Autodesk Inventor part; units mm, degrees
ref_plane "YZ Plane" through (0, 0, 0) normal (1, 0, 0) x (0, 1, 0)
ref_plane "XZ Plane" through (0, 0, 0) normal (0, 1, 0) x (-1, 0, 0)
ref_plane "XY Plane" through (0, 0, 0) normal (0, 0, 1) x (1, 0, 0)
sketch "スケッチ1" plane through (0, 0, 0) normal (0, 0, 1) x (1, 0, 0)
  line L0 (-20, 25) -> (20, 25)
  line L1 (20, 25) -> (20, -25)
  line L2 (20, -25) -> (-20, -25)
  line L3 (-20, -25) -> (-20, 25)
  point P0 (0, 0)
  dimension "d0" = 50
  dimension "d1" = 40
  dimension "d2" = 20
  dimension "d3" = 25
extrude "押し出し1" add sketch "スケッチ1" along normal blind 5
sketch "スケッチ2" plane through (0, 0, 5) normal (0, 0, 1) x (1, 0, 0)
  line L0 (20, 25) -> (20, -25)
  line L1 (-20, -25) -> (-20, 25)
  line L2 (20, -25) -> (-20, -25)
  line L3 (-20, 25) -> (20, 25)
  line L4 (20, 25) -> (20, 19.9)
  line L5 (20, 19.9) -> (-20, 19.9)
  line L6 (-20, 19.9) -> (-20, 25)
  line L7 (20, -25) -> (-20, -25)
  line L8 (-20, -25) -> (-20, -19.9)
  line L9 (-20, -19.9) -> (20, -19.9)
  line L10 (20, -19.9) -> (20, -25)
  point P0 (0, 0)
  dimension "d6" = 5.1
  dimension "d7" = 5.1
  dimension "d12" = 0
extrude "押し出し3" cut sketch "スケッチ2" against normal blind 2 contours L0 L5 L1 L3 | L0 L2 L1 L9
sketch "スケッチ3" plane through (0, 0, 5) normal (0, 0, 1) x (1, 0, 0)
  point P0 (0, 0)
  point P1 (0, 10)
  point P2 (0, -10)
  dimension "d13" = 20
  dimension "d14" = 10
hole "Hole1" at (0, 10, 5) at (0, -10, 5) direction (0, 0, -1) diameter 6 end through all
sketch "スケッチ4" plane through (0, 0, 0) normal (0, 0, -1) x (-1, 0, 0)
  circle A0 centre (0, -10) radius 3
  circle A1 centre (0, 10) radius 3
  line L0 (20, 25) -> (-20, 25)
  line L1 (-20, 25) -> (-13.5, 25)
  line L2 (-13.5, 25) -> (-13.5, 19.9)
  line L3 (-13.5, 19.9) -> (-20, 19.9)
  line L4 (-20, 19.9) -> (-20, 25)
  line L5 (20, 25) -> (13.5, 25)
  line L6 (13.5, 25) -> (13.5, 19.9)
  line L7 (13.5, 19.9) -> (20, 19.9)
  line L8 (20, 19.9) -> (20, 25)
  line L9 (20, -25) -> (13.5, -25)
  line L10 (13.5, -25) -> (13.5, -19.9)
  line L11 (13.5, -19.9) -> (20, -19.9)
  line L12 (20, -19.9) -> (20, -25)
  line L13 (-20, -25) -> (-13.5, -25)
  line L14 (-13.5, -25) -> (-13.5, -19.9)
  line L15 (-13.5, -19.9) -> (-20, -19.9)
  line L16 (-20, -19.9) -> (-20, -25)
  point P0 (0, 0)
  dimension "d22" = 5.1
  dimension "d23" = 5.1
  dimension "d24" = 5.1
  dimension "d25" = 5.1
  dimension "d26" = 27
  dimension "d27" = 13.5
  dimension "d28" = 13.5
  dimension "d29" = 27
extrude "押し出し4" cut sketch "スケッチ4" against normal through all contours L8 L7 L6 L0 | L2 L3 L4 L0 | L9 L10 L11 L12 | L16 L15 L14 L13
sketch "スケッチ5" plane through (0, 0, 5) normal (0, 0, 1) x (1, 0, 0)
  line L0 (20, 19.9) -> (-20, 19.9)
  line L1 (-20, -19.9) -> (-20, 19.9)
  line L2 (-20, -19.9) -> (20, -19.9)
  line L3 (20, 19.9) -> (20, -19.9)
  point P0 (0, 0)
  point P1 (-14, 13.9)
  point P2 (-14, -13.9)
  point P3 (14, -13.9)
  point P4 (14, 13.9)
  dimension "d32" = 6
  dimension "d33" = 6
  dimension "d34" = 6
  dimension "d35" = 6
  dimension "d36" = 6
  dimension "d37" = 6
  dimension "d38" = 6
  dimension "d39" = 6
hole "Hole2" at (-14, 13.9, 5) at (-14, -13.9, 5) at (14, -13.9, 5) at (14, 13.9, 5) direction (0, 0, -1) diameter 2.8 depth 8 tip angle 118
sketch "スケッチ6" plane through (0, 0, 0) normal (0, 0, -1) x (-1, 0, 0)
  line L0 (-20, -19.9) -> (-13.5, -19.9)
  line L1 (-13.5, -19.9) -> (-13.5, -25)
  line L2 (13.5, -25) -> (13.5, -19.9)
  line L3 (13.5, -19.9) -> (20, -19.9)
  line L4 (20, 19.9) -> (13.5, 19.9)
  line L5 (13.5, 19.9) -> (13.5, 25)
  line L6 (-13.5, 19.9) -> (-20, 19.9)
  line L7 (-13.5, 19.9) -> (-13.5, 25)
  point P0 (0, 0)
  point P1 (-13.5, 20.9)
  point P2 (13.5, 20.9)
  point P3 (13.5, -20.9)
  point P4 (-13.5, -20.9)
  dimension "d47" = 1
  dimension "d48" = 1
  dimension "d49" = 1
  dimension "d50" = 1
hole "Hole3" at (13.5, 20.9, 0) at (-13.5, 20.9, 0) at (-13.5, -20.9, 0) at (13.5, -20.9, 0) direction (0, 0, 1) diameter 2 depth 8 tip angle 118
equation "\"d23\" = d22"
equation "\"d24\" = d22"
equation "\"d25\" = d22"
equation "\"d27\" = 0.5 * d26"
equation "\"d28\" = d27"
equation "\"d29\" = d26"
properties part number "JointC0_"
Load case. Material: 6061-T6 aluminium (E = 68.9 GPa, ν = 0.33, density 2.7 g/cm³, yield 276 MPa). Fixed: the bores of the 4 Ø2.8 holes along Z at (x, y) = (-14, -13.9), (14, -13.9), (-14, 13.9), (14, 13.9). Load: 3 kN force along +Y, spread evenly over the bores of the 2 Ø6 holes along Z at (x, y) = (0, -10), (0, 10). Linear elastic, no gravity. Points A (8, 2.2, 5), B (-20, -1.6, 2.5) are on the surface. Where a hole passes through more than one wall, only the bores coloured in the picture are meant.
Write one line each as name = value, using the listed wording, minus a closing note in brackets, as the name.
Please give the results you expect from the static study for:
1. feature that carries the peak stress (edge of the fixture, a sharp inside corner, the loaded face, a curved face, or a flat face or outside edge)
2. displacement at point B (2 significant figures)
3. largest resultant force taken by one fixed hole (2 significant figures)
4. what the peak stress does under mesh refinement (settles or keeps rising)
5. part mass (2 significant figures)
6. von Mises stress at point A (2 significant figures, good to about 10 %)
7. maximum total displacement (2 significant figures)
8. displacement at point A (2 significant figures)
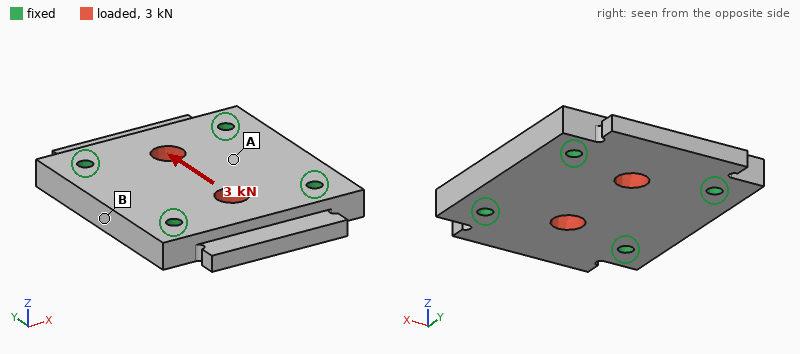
feature that carries the peak stress = edge of the fixture
displacement at point B = 0.75 µm
largest resultant force taken by one fixed hole = 770 N
what the peak stress does under mesh refinement = keeps rising
part mass = 23 g
von Mises stress at point A = 13 MPa
maximum total displacement = 5.0 µm
displacement at point A = 2.5 µm
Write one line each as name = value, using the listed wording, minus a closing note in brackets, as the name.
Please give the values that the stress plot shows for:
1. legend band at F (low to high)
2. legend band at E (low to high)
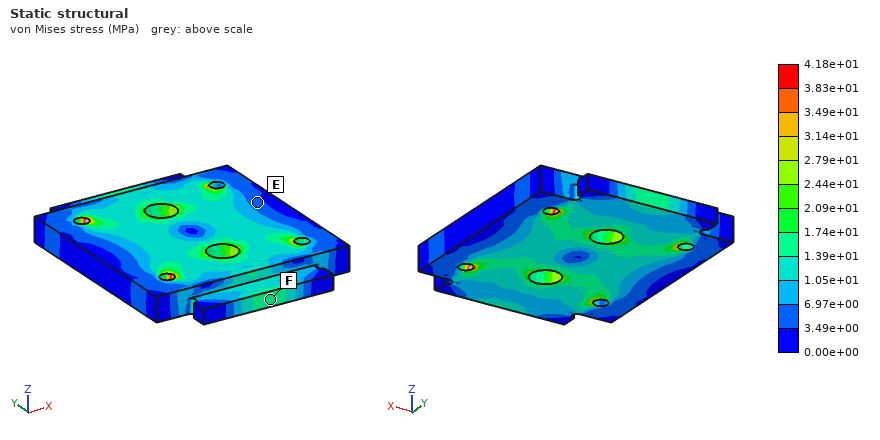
legend band at F = 1.39e+01 to 1.74e+01 MPa
legend band at E = 3.49e+00 to 6.97e+00 MPa
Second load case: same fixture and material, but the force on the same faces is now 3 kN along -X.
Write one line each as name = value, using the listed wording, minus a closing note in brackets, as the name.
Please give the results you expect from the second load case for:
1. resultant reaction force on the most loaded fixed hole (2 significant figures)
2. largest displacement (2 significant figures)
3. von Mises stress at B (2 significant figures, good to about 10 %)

resultant reaction force on the most loaded fixed hole = 770 N
largest displacement = 3.5 µm
von Mises stress at B = 7.0 MPa
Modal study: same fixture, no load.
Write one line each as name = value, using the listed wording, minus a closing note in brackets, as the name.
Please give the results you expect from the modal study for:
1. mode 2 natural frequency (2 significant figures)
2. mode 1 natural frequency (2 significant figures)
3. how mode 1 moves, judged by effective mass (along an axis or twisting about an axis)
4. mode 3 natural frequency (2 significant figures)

mode 2 natural frequency = 21 kHz
mode 1 natural frequency = 20 kHz
how mode 1 moves, judged by effective mass = along Z
mode 3 natural frequency = 21 kHz
